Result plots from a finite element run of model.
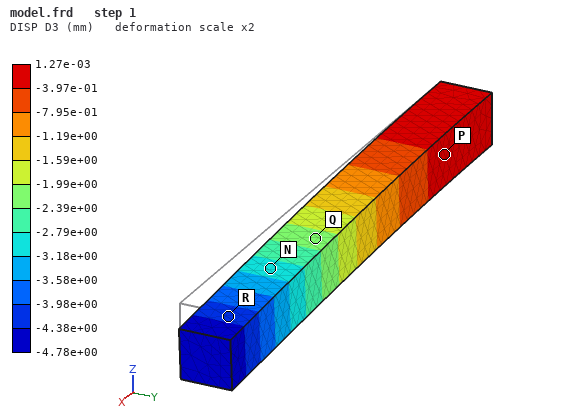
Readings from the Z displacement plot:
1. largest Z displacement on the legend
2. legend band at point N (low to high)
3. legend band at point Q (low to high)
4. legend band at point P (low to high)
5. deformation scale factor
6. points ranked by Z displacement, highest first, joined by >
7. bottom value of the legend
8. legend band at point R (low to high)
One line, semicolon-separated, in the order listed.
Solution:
1.27e-03 mm; -3.18e+00 to -2.79e+00 mm; -2.39e+00 to -1.99e+00 mm; -3.97e-01 to 1.27e-03 mm; 2; P > Q > N > R; -4.78e+00 mm; -4.38e+00 to -3.98e+00 mm
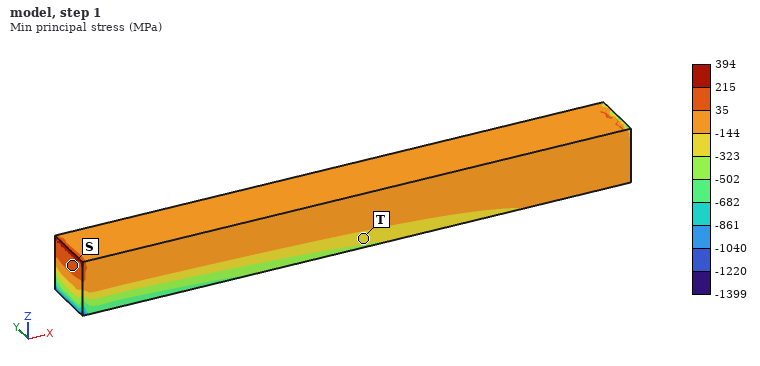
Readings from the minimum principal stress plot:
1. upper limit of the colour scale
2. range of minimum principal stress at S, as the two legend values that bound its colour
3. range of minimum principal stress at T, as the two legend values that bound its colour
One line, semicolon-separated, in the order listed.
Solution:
394 MPa; 35 to 215 MPa; -323 to -144 MPa
